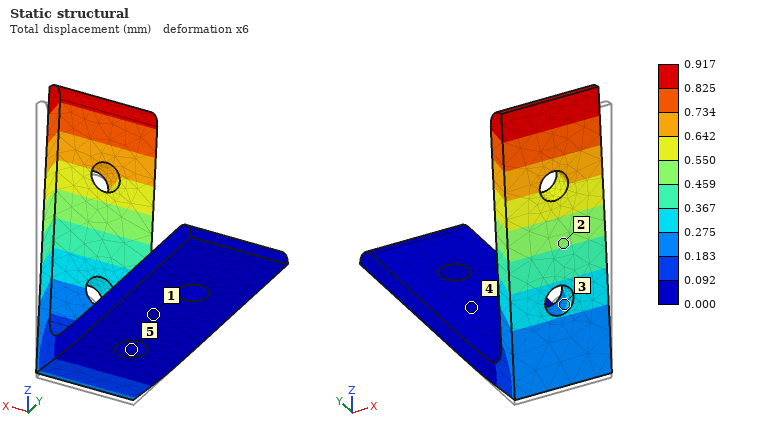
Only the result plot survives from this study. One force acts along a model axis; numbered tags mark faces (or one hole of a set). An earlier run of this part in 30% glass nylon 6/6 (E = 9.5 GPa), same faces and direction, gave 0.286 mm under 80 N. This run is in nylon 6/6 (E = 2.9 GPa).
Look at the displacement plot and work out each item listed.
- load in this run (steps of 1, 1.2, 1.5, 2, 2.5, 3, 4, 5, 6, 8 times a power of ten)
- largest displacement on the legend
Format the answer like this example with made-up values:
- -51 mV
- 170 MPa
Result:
- 80 N
- 0.917 mm
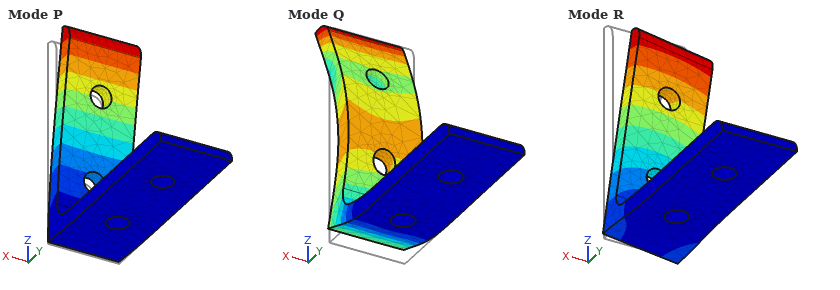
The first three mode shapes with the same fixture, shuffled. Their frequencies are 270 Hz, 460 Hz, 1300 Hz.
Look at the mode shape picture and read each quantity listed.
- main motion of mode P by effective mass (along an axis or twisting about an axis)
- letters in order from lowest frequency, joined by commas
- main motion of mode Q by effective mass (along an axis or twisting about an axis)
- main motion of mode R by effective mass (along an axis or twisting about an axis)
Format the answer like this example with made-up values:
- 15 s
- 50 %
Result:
- along Y
- P, R, Q
- along Z
- along X
